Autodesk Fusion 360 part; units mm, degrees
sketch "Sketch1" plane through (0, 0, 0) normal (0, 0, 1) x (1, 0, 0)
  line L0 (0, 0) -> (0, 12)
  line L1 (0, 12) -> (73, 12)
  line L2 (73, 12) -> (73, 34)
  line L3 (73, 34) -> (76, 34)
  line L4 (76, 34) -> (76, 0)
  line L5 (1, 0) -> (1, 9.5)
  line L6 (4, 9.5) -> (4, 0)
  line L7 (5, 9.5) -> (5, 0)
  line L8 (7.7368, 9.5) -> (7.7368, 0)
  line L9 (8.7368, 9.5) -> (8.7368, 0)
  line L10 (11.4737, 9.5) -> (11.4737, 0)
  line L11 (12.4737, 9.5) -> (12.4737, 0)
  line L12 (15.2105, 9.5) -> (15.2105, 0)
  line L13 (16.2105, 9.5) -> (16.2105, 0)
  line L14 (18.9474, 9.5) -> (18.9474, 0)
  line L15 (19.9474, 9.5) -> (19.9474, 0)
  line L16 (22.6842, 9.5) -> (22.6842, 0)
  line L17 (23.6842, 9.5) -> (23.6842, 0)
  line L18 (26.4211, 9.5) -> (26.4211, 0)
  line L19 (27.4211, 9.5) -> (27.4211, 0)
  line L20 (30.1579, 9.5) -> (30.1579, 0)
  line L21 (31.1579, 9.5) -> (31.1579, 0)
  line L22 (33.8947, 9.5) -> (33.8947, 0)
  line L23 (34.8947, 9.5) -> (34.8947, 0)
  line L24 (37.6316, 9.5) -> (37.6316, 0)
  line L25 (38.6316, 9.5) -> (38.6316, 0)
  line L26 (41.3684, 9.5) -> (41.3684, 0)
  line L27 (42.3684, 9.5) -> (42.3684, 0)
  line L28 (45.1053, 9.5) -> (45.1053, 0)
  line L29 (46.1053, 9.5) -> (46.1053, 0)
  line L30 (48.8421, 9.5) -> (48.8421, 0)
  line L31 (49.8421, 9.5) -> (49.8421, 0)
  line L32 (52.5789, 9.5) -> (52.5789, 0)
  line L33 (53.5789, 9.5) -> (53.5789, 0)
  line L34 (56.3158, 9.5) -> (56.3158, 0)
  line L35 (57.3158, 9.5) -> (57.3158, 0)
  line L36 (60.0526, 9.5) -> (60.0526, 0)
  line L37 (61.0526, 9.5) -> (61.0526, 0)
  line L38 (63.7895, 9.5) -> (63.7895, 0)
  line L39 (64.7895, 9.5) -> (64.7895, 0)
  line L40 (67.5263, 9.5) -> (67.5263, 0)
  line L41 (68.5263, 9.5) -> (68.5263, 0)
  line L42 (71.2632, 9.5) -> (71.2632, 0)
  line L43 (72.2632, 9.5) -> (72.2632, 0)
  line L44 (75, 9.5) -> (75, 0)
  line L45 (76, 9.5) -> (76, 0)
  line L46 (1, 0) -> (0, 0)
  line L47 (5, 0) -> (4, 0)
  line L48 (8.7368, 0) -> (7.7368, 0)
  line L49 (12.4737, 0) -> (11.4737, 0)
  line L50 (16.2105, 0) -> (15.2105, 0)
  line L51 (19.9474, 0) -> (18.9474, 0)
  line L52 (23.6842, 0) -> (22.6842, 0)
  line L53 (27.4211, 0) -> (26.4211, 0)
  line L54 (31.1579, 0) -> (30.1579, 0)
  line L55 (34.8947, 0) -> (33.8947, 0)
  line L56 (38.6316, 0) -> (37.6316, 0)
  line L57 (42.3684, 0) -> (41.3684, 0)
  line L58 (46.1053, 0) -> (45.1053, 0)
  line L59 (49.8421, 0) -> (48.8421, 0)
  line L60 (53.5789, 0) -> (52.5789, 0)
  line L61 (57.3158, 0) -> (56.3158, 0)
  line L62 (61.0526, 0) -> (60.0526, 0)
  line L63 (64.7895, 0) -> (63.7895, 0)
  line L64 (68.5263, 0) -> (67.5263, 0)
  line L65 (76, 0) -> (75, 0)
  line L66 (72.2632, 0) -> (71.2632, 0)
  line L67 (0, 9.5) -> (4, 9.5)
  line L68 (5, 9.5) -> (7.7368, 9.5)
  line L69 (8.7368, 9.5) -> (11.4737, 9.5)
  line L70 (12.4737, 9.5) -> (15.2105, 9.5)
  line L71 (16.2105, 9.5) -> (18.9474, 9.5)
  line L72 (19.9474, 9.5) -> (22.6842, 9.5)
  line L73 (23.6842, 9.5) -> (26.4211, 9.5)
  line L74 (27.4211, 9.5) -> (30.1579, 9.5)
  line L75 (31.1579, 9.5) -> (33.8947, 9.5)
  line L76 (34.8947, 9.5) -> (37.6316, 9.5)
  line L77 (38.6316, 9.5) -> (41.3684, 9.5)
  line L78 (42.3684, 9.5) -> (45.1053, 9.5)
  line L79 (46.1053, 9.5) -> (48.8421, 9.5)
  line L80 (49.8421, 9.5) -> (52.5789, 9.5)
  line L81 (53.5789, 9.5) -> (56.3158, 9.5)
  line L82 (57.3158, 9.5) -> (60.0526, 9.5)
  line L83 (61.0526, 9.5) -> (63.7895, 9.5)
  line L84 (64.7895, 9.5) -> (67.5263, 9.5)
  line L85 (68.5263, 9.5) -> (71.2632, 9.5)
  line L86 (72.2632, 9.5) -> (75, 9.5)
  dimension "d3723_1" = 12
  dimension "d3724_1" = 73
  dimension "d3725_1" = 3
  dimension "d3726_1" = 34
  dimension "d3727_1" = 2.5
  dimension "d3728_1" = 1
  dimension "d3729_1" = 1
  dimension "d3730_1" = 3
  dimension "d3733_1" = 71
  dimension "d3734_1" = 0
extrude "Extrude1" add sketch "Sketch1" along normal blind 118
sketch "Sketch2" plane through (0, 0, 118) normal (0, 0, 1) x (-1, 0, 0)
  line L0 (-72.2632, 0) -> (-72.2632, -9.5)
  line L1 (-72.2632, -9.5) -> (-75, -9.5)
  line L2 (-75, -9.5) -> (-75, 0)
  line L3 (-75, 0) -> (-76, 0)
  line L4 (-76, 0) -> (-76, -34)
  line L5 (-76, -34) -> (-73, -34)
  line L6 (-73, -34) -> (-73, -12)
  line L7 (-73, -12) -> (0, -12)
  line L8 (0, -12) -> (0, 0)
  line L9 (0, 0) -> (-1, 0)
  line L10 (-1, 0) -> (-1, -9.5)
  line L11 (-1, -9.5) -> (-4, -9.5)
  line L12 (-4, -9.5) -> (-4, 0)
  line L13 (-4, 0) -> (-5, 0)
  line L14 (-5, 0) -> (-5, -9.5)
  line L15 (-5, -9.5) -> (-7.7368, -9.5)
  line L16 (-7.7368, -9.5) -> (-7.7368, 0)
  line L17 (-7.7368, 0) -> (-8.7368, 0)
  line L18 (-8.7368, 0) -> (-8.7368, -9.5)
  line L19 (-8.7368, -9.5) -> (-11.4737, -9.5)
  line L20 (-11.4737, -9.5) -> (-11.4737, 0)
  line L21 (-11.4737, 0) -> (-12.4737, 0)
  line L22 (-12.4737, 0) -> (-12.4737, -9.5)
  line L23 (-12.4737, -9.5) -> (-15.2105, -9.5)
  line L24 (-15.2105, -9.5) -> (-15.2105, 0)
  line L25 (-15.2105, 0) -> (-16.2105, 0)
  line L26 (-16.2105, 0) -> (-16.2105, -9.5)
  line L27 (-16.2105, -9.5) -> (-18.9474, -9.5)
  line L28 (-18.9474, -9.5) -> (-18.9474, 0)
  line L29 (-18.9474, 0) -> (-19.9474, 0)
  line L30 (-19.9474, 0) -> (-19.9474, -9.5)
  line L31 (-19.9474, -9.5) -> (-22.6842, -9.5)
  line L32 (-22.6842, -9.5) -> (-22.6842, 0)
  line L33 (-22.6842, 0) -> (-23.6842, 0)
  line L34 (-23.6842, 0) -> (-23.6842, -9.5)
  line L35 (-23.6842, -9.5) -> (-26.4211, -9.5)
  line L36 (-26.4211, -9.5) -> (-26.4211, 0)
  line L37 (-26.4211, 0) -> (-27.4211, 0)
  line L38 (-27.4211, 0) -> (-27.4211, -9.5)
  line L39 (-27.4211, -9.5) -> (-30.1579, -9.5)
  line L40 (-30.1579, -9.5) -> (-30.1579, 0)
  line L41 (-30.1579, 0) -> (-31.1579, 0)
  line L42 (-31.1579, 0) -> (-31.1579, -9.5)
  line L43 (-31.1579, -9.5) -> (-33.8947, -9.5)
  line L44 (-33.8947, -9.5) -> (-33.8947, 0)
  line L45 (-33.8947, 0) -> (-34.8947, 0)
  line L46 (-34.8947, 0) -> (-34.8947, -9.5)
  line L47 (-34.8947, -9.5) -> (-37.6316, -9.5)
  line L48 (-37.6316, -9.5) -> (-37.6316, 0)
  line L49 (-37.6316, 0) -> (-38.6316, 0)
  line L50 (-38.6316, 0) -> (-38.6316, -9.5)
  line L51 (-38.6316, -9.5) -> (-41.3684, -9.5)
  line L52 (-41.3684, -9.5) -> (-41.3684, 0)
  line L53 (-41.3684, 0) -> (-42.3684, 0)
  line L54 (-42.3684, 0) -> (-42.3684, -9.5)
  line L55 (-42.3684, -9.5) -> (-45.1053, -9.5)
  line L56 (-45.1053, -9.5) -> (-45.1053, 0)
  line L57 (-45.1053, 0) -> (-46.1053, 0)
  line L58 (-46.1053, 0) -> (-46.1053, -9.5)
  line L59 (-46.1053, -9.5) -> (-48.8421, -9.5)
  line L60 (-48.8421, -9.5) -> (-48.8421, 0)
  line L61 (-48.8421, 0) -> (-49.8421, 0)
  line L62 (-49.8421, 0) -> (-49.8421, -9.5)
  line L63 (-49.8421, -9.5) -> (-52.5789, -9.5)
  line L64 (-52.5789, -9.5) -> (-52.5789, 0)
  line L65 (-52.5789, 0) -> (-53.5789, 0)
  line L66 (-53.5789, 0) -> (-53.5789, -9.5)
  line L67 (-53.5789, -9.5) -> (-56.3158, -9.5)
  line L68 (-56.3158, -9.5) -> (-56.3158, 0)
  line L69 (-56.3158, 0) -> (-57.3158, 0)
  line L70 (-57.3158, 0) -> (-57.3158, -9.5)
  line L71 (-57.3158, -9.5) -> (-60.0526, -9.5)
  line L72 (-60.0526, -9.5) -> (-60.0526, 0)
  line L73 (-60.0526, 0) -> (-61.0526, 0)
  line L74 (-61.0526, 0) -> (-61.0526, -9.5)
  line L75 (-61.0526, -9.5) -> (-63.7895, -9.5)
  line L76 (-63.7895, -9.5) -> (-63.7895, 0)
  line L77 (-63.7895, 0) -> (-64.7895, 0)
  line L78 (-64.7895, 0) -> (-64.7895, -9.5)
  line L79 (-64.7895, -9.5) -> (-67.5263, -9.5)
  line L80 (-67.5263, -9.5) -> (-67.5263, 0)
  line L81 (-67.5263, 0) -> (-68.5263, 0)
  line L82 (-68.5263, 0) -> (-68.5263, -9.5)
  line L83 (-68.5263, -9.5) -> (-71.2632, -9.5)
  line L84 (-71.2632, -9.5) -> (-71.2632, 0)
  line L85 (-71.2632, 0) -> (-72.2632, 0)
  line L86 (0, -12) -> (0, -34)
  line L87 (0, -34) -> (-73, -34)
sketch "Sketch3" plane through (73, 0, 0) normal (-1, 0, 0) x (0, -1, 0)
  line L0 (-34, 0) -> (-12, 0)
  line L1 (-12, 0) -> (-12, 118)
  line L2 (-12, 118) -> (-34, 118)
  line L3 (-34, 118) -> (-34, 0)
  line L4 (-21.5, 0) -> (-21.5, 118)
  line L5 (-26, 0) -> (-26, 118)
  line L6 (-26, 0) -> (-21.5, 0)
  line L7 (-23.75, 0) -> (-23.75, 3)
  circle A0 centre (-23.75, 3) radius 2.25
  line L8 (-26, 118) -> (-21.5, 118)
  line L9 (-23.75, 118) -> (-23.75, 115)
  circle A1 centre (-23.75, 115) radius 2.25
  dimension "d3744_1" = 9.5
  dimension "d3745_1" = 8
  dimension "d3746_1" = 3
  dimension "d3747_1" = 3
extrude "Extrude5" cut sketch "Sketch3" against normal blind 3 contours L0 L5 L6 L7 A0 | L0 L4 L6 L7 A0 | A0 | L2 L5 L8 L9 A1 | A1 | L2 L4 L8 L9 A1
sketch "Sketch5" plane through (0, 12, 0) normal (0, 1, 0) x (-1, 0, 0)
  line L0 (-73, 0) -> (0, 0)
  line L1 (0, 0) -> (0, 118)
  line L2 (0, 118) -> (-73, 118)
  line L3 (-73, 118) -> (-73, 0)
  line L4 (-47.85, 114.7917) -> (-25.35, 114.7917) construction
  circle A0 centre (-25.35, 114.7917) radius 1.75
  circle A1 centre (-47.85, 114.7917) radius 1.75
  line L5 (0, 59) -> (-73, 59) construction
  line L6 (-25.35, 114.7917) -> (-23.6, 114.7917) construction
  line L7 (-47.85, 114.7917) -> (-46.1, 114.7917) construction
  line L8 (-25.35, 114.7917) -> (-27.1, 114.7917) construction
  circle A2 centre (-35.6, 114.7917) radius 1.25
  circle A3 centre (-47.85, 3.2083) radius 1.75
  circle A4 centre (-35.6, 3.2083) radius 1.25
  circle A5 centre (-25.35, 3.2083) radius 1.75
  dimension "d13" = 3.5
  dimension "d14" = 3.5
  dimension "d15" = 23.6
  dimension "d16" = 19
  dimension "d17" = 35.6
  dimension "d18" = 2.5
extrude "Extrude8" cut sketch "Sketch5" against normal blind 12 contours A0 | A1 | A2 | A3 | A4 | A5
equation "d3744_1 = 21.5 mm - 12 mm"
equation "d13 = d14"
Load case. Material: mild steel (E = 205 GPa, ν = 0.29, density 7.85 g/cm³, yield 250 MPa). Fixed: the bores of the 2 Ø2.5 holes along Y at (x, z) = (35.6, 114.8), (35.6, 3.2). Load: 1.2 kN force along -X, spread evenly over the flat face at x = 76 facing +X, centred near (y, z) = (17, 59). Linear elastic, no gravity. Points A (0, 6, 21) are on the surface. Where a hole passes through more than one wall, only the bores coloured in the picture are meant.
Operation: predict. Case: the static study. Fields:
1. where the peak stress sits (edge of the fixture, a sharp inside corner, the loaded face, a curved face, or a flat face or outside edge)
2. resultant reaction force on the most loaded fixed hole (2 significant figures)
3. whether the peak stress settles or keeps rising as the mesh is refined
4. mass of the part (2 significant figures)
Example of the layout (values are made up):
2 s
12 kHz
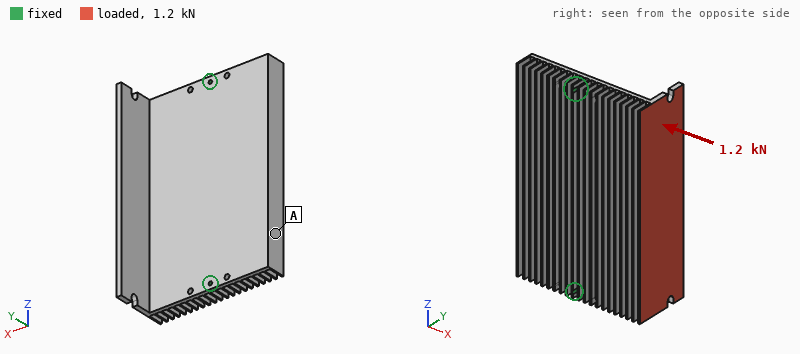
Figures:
edge of the fixture
620 N
keeps rising
420 g
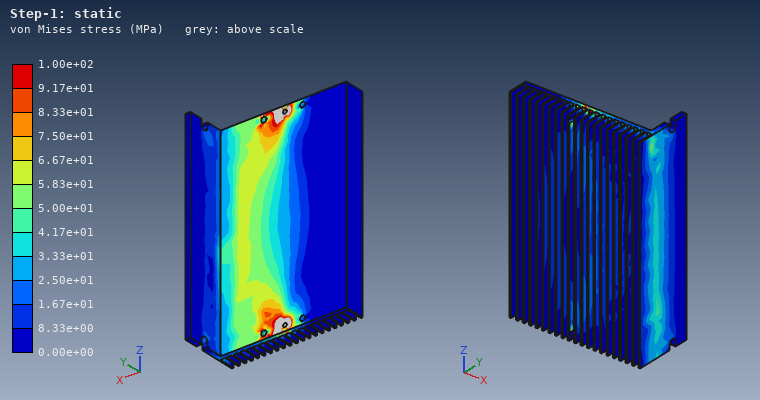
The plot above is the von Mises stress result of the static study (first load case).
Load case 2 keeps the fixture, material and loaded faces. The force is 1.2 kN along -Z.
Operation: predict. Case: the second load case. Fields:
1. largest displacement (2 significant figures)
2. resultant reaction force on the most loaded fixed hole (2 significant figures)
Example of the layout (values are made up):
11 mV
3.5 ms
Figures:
0.10 mm
750 N
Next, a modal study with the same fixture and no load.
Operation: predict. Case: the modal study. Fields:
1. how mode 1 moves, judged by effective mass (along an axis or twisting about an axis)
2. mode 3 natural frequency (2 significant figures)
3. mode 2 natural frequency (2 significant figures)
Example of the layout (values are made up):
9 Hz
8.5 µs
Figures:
along Y
910 Hz
870 Hz
